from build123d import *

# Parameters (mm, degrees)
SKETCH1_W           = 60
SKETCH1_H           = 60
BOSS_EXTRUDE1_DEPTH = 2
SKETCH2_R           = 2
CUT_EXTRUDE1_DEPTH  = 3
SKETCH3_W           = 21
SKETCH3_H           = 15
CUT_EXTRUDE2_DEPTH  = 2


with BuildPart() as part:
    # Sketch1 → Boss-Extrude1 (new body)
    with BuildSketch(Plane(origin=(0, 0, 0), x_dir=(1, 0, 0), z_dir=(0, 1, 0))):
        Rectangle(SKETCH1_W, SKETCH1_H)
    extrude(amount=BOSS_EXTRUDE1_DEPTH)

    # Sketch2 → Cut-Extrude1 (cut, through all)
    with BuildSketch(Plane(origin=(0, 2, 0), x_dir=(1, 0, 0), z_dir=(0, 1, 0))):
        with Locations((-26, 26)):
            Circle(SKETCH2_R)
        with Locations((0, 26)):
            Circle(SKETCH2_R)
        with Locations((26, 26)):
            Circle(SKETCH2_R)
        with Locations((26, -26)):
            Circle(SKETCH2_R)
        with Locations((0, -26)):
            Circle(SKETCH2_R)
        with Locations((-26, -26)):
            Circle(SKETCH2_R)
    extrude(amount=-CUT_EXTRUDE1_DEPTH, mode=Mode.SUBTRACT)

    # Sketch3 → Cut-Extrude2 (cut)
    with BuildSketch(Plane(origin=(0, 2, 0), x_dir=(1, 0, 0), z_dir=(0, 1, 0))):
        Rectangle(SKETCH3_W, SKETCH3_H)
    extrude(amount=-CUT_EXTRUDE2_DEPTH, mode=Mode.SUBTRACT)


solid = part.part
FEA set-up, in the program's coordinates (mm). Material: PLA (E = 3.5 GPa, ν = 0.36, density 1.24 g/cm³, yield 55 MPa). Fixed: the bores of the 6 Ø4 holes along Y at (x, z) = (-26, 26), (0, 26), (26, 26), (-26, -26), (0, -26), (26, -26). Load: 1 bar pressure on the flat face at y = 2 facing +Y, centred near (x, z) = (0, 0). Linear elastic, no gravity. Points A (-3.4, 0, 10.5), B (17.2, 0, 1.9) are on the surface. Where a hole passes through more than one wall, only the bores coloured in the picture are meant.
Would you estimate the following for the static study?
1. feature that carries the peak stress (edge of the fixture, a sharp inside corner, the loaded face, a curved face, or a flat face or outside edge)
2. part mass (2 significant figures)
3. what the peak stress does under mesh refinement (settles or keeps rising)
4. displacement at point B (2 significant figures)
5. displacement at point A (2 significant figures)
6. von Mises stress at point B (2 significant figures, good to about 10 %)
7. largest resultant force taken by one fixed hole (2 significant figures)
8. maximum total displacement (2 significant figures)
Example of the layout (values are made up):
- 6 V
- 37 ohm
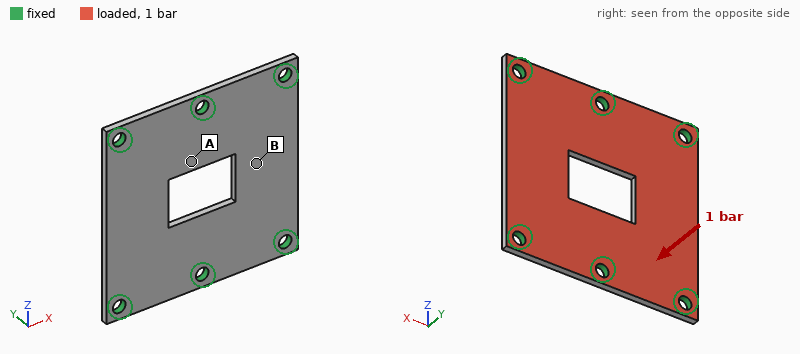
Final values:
- edge of the fixture
- 8.0 g
- keeps rising
- 0.78 mm
- 0.59 mm
- 15 MPa
- 68 N
- 0.86 mm
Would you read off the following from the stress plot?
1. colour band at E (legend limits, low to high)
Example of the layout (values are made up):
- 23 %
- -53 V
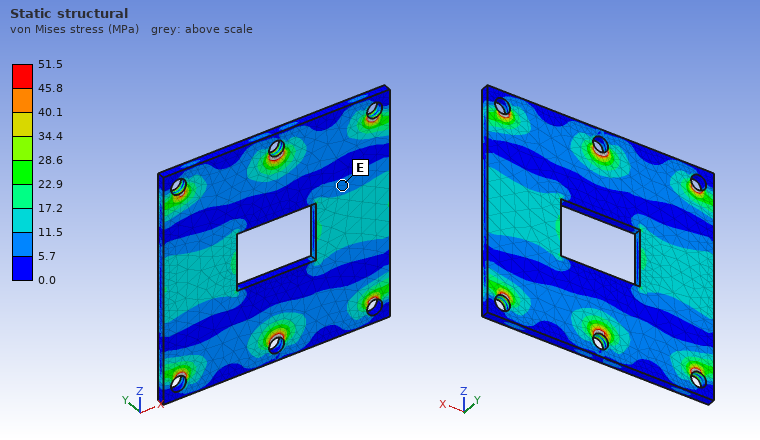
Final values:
- 5.7 to 11.5 MPa
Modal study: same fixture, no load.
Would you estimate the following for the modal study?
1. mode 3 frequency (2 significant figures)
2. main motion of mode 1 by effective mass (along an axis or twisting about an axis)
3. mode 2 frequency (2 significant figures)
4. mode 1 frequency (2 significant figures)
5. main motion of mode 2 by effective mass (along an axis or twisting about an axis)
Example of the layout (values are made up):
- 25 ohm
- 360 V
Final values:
- 2400 Hz
- along Y
- 1500 Hz
- 1300 Hz
- twisting about Z
